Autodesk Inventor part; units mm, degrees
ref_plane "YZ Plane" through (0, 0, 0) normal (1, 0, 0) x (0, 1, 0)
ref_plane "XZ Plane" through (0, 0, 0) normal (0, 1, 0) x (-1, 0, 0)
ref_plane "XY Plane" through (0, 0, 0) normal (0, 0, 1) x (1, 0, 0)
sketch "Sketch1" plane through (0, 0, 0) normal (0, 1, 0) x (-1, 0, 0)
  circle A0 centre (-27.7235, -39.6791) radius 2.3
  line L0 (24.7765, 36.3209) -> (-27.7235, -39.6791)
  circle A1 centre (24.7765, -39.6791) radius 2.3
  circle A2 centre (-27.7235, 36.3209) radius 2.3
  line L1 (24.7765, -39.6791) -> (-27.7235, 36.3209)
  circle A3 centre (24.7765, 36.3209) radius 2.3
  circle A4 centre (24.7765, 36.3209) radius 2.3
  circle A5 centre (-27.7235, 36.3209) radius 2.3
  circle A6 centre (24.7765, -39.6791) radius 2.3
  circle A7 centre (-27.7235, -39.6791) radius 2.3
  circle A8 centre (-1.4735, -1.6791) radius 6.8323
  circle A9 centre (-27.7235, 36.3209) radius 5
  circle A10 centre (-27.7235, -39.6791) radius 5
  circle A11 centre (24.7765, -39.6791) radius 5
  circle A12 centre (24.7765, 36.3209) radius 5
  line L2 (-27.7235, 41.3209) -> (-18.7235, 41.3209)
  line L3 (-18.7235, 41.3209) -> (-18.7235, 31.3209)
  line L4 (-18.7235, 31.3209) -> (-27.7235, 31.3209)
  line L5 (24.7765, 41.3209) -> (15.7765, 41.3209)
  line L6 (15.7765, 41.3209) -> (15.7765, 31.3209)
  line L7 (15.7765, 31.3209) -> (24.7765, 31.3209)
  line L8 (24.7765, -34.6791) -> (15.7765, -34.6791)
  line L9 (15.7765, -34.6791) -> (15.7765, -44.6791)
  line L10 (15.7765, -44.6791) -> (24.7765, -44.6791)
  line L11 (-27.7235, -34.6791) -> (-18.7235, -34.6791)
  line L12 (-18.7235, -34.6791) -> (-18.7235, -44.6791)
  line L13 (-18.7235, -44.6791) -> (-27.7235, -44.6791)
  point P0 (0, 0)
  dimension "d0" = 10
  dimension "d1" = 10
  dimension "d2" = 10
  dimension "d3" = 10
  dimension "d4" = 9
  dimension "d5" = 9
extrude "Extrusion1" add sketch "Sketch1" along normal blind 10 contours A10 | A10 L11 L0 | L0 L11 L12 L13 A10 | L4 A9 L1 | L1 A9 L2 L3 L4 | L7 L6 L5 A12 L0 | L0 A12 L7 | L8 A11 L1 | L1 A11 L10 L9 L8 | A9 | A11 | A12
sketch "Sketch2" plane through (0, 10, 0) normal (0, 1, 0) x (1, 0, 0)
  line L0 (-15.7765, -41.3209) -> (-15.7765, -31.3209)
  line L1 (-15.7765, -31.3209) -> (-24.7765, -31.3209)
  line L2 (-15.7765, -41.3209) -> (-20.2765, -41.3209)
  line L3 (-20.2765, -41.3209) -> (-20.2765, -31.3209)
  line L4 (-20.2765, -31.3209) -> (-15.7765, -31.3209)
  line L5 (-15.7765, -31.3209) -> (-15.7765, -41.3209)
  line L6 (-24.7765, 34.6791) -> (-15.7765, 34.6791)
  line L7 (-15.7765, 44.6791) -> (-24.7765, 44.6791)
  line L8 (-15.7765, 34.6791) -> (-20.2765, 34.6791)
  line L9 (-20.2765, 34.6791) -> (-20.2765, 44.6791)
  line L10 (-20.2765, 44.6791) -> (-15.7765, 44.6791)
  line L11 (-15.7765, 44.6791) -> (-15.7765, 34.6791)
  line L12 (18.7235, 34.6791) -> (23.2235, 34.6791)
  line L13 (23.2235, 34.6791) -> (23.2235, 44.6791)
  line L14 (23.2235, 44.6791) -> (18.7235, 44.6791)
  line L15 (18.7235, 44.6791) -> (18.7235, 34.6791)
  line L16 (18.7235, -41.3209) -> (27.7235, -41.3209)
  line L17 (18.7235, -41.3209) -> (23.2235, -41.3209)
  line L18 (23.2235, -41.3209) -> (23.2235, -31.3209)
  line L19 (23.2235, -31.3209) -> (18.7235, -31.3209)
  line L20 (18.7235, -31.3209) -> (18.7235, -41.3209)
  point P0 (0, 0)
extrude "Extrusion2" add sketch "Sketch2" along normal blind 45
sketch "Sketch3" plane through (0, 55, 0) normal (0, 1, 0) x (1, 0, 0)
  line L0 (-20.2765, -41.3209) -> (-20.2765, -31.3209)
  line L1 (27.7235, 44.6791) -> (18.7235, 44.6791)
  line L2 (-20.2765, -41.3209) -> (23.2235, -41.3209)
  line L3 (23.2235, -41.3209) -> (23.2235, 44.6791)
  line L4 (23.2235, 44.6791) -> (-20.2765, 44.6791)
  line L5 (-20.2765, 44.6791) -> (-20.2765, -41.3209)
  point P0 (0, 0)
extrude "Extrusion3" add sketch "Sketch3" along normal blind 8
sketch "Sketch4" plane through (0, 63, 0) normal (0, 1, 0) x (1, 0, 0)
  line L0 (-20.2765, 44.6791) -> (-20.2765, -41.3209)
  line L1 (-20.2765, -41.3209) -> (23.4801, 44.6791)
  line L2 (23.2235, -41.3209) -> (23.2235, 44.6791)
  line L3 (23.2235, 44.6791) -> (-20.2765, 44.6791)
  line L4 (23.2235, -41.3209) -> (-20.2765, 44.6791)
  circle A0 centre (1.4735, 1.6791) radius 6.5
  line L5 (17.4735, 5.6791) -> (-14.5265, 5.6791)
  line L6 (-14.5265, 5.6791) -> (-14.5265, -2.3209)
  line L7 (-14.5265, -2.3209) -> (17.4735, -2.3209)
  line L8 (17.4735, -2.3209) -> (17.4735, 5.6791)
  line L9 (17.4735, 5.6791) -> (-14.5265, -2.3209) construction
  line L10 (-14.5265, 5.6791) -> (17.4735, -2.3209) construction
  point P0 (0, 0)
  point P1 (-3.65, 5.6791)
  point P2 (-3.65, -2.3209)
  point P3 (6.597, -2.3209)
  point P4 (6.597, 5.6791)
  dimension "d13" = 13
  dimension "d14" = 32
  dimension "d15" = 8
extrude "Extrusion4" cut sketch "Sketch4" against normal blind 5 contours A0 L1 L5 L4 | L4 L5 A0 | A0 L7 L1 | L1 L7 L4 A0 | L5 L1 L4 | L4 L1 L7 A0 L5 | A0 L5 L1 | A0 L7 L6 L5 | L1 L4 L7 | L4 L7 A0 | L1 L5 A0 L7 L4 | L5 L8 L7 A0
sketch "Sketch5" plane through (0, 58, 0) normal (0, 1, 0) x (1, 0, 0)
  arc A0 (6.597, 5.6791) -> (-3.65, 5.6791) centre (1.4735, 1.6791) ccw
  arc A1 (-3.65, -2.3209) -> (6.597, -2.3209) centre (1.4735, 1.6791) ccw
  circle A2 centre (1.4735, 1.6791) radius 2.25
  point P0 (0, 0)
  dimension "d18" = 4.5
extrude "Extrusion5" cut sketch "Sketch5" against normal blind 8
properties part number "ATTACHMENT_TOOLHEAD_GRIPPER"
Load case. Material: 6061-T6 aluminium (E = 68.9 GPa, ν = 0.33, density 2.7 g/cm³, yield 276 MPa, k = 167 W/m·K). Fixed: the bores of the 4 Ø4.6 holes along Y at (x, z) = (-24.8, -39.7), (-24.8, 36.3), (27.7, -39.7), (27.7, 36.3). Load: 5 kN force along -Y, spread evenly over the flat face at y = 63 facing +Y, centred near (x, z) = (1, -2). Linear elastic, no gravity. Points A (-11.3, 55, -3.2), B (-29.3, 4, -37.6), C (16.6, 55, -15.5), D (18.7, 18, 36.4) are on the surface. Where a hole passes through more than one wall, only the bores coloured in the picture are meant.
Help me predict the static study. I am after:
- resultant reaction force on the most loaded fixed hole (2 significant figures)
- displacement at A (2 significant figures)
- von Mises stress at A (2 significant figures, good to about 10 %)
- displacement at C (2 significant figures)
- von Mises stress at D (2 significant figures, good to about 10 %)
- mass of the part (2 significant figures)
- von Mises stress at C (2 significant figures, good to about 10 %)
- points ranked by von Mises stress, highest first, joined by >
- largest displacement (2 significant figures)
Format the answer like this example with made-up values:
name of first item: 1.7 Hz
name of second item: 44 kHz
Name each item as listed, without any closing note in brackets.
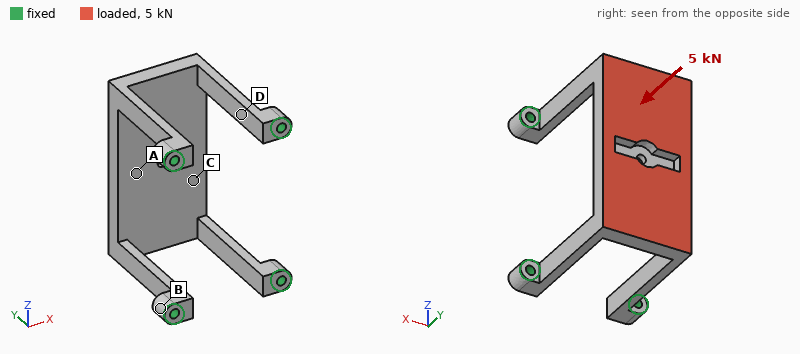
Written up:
resultant reaction force on the most loaded fixed hole: 1.3 kN
displacement at A: 0.18 mm
von Mises stress at A: 69 MPa
displacement at C: 0.15 mm
von Mises stress at D: 21 MPa
mass of the part: 110 g
von Mises stress at C: 38 MPa
points ranked by von Mises stress, highest first, joined by >: A > C > D > B
largest displacement: 0.19 mm
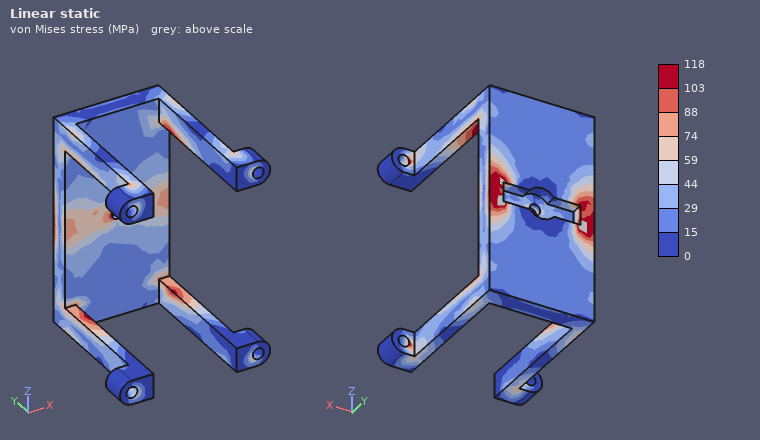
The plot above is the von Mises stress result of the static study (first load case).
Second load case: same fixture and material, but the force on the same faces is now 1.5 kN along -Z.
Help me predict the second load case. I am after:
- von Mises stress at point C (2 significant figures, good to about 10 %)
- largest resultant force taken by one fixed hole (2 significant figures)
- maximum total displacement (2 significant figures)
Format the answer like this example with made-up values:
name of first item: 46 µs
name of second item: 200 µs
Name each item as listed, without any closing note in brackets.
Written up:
von Mises stress at point C: 20 MPa
largest resultant force taken by one fixed hole: 470 N
maximum total displacement: 0.29 mm
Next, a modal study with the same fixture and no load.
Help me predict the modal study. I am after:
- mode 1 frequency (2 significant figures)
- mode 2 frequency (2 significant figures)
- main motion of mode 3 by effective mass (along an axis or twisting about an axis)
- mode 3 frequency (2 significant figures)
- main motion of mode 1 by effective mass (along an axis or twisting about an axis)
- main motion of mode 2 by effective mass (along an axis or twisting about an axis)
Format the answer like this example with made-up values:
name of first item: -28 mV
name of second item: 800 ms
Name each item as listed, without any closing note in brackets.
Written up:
mode 1 frequency: 780 Hz
mode 2 frequency: 1300 Hz
main motion of mode 3 by effective mass: twisting about Y
mode 3 frequency: 1400 Hz
main motion of mode 1 by effective mass: along X
main motion of mode 2 by effective mass: along Z
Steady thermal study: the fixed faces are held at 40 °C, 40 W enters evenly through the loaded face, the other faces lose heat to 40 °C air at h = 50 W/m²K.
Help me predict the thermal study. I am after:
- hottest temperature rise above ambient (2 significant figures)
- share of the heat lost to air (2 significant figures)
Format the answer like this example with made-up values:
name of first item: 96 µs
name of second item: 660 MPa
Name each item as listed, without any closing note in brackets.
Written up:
hottest temperature rise above ambient: 44 K
share of the heat lost to air: 47 %
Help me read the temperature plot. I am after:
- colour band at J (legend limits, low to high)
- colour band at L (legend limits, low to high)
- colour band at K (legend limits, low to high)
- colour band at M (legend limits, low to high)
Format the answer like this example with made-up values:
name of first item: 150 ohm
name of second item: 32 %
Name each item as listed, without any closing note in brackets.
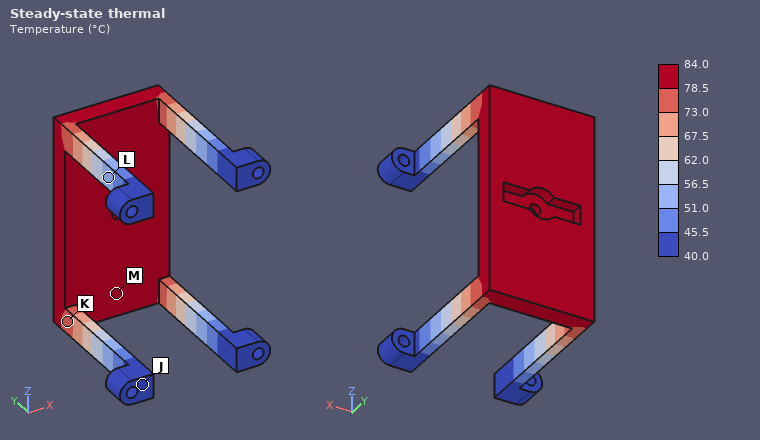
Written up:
colour band at J: 40.0 to 45.5 °C
colour band at L: 51.0 to 56.5 °C
colour band at K: 73.0 to 78.5 °C
colour band at M: 78.5 to 84.0 °C
